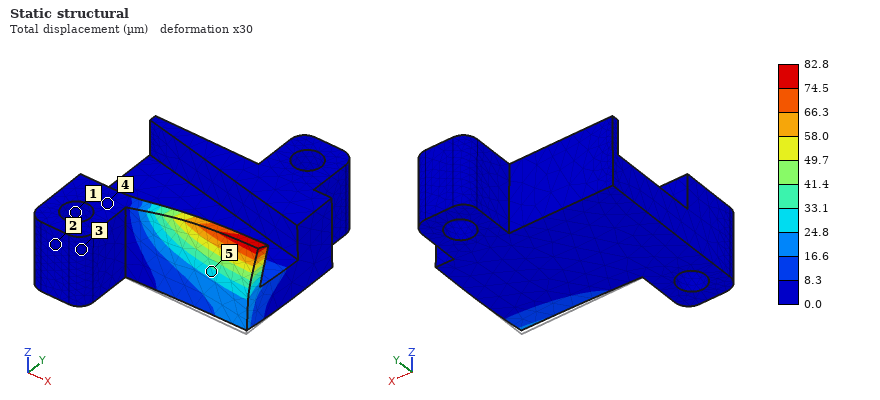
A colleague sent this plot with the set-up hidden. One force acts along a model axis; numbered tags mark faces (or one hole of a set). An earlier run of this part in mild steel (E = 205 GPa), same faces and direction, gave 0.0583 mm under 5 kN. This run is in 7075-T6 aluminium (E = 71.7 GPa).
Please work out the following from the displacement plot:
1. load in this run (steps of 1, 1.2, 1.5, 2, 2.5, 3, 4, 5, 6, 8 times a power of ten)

2.5 kN
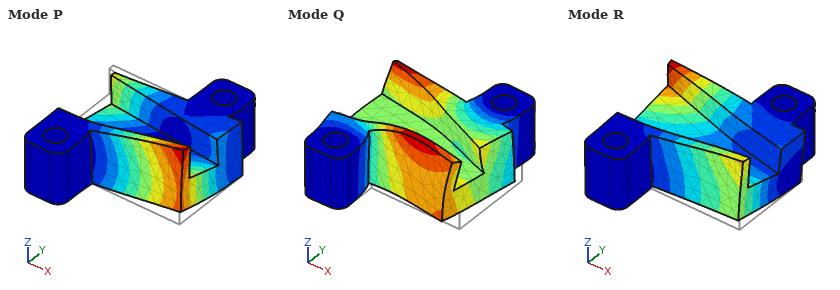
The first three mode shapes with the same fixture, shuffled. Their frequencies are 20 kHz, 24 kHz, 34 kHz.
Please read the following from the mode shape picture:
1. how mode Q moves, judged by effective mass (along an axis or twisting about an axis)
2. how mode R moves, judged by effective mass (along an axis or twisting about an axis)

along X
along Z
